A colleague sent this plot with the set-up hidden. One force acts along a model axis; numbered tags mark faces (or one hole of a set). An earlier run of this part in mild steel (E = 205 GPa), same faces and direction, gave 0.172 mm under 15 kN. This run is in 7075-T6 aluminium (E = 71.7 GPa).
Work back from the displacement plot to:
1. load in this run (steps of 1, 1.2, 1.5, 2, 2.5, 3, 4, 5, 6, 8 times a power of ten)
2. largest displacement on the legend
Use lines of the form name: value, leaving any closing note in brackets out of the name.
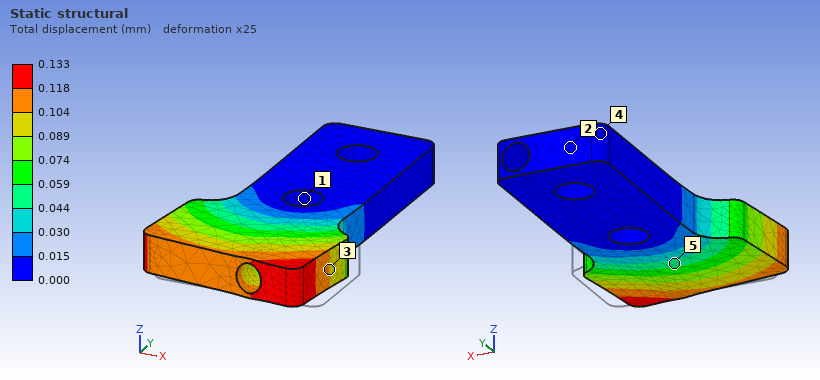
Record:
load in this run: 4 kN
largest displacement on the legend: 0.133 mm
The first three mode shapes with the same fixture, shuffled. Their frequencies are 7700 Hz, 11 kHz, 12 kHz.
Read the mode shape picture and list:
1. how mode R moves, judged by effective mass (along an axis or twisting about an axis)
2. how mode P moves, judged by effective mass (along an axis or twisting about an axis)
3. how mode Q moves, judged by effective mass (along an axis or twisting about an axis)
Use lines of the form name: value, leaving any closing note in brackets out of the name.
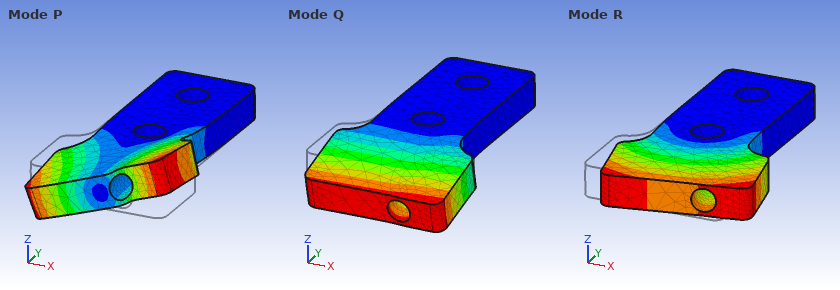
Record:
how mode R moves, judged by effective mass: along X
how mode P moves, judged by effective mass: twisting about Y
how mode Q moves, judged by effective mass: along Z
